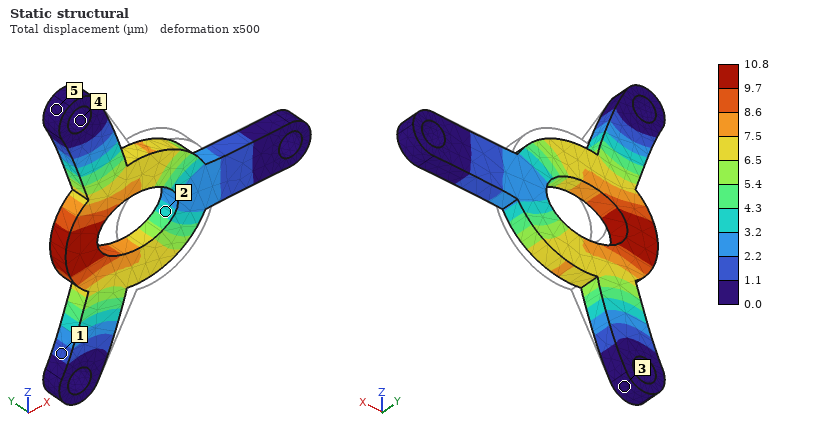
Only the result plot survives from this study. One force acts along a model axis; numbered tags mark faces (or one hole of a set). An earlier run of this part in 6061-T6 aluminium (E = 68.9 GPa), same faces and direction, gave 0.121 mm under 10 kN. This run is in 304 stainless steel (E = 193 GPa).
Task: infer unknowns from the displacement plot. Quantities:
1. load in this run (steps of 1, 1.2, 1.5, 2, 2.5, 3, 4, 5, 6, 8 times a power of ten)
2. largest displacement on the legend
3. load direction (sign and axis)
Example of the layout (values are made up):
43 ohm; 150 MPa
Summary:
2.5 kN; 10.8 µm; -X
